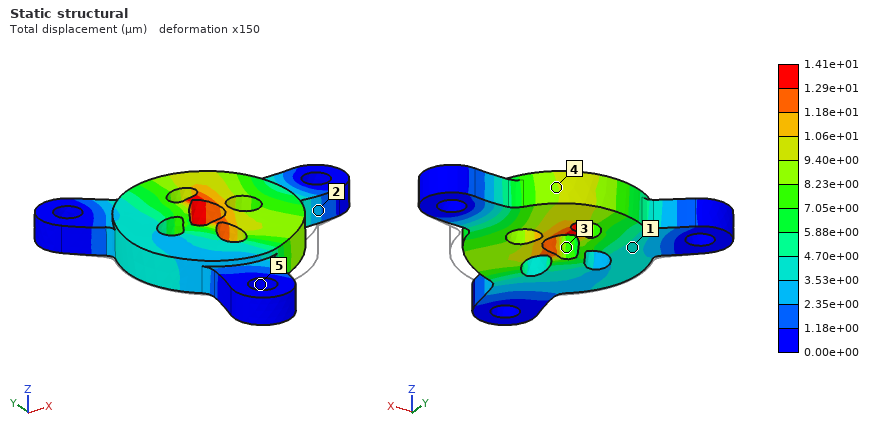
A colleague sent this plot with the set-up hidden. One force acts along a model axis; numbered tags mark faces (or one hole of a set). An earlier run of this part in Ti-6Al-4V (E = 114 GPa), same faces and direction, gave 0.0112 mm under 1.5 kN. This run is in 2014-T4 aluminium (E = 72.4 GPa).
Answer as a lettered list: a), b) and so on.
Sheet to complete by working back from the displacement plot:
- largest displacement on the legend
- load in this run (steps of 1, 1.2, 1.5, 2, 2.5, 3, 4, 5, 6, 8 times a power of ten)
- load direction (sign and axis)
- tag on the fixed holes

a) 1.41e+01 µm
b) 1.2 kN
c) +Y
d) 5
